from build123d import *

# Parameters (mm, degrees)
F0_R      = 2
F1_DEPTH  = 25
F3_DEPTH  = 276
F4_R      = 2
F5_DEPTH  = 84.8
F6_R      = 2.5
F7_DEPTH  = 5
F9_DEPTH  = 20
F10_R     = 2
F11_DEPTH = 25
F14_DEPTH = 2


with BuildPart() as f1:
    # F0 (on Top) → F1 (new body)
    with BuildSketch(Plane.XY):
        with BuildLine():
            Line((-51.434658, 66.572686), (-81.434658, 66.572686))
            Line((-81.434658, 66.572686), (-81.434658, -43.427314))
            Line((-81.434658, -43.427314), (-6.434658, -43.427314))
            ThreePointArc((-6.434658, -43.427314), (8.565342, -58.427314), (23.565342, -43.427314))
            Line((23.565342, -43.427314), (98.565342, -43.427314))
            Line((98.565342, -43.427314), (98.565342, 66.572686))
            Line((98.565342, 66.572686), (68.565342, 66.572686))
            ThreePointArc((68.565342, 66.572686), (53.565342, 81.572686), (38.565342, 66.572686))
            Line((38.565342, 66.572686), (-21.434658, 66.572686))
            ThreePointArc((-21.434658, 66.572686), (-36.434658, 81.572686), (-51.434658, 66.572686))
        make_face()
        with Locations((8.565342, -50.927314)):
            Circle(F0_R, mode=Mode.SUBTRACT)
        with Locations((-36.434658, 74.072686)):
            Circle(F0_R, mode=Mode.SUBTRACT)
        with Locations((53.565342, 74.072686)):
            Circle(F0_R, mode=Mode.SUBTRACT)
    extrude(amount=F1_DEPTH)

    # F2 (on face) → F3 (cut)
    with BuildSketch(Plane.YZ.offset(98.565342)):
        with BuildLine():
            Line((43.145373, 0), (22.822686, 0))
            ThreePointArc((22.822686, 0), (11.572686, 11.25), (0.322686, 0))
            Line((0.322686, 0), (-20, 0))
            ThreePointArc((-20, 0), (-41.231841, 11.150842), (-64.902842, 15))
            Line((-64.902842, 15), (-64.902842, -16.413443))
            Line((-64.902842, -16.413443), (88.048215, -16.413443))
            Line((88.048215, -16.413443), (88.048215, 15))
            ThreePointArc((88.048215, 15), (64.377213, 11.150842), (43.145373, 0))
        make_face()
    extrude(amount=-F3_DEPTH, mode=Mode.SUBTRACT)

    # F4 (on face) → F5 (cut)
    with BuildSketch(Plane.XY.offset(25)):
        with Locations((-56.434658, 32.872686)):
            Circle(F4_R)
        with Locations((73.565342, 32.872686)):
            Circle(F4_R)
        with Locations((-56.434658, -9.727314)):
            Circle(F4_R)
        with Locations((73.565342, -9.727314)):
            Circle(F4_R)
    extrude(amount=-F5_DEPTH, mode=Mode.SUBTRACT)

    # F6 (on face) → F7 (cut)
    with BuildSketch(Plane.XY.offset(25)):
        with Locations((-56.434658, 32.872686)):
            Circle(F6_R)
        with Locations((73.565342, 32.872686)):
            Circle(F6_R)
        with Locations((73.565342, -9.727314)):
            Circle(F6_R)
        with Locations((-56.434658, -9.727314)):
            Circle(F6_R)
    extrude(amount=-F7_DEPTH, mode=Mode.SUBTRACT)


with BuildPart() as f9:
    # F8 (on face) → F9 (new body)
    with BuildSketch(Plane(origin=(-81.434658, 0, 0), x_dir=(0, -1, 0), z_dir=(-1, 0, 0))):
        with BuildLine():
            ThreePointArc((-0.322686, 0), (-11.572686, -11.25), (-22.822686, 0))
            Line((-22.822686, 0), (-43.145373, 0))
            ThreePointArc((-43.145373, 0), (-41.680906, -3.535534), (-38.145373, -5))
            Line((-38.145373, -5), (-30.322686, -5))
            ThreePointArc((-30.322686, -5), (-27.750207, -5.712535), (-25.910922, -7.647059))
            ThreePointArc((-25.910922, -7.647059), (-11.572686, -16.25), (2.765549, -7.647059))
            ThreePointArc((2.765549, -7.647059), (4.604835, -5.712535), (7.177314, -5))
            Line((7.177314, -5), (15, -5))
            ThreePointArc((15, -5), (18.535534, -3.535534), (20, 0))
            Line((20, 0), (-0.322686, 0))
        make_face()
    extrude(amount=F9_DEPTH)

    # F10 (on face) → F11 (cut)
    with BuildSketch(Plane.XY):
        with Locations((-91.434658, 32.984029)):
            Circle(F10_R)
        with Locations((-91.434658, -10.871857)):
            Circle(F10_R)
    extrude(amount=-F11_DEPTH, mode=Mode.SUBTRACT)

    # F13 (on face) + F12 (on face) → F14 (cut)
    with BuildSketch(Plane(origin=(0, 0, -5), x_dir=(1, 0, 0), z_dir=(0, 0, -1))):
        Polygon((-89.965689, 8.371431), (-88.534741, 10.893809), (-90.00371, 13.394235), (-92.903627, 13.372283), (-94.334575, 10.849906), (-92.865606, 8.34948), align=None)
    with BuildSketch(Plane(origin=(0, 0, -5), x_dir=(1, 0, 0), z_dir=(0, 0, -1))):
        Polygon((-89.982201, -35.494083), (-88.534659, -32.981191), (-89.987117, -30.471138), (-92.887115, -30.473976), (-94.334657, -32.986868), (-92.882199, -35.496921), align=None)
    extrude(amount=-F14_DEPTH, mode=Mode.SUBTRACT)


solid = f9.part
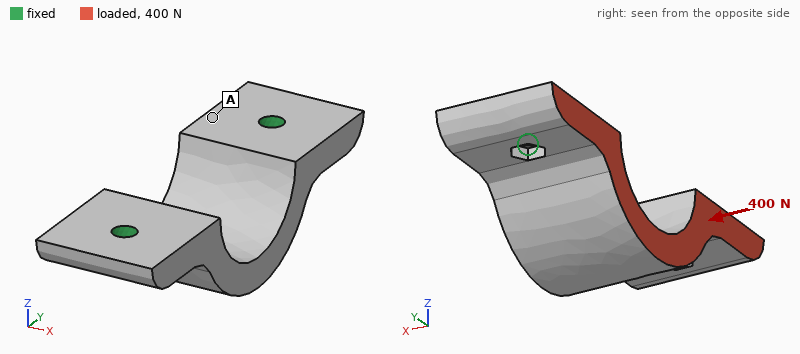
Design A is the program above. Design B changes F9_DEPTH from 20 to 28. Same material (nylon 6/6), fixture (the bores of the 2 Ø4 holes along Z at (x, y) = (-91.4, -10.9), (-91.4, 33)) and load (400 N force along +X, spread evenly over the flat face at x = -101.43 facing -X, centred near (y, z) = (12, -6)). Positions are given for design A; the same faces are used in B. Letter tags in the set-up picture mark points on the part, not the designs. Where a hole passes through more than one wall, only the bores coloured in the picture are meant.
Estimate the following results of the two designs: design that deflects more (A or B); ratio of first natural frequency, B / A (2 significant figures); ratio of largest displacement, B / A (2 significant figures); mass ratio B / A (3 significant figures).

B
0.72
1.2
1.41
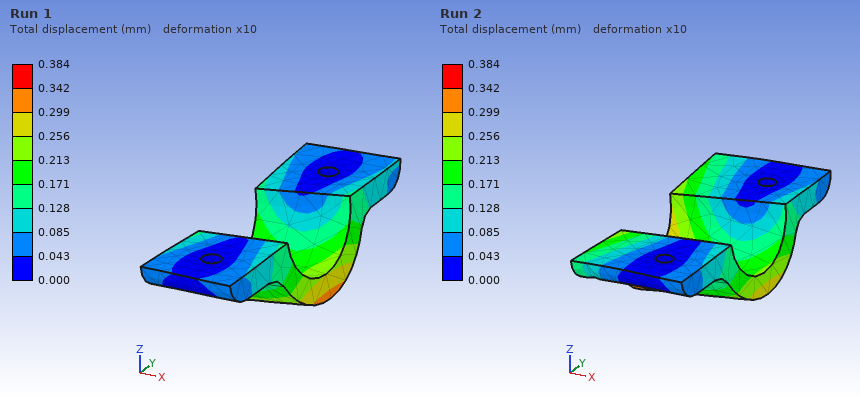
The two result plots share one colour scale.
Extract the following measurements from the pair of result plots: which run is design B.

Run 2
